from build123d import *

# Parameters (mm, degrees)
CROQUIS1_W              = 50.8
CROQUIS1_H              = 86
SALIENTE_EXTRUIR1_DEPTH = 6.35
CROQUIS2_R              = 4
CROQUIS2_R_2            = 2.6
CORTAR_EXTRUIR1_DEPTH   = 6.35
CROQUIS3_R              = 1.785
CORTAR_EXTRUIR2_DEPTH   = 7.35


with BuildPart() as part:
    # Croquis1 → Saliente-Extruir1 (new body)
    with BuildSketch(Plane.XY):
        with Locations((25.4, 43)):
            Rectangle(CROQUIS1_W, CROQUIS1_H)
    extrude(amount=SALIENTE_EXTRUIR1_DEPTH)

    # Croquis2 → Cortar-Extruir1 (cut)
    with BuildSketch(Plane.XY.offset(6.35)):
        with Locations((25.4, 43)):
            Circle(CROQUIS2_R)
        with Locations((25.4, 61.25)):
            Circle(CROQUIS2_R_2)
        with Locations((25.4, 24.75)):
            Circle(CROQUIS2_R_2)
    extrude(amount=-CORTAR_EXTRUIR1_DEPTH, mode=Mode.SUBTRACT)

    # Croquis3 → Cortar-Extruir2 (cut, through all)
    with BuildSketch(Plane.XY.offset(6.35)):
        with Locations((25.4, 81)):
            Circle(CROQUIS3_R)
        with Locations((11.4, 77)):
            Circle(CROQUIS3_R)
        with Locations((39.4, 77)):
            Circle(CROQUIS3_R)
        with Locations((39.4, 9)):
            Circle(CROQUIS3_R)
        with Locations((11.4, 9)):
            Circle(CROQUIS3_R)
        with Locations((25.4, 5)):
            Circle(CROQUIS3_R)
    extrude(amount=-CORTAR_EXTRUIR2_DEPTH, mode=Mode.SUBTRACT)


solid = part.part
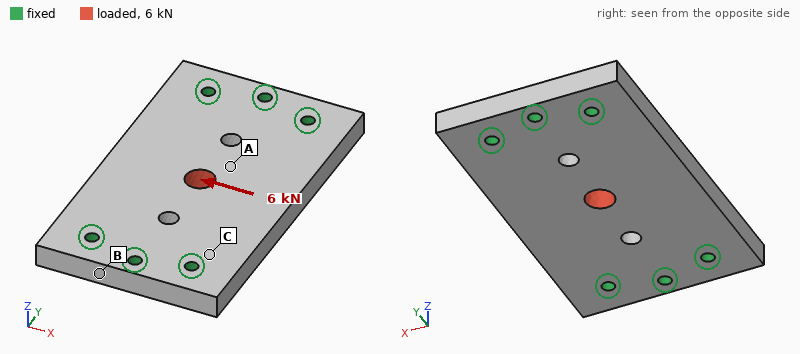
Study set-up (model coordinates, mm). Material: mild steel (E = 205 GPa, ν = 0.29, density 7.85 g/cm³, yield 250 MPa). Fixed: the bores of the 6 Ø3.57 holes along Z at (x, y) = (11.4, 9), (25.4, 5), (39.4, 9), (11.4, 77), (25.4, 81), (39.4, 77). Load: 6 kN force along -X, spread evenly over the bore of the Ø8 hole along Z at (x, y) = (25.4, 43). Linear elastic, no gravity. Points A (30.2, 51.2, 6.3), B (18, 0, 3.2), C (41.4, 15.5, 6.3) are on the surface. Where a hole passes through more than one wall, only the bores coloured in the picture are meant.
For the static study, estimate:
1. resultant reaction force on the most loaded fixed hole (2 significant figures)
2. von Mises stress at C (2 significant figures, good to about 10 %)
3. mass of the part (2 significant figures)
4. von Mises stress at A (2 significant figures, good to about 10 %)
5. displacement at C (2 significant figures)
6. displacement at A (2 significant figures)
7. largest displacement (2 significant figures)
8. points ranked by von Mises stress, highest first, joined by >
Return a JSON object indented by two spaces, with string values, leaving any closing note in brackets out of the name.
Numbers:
{
  "resultant reaction force on the most loaded fixed hole": "1.8 kN",
  "von Mises stress at C": "14 MPa",
  "mass of the part": "210 g",
  "von Mises stress at A": "24 MPa",
  "displacement at C": "1.4 µm",
  "displacement at A": "5.3 µm",
  "largest displacement": "6.9 µm",
  "points ranked by von Mises stress, highest first, joined by >": "A > C > B"
}
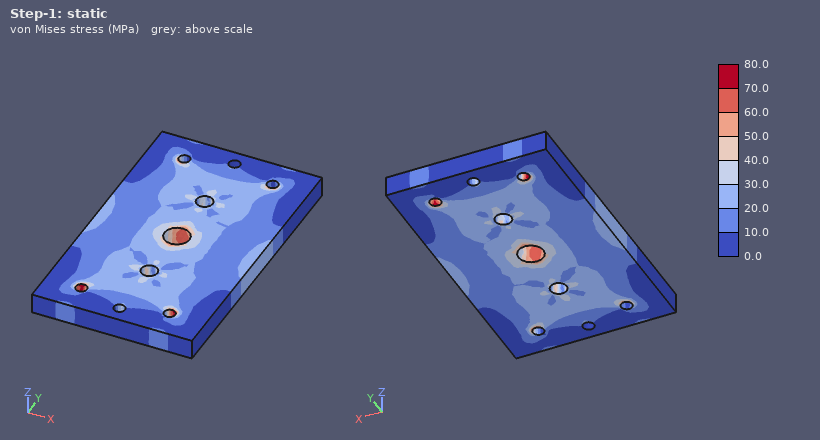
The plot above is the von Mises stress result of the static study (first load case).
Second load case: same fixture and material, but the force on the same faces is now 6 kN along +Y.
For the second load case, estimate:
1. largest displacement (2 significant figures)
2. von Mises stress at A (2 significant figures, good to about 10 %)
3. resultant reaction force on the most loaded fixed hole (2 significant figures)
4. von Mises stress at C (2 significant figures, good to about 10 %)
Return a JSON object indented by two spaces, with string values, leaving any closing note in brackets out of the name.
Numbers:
{
  "largest displacement": "3.3 µm",
  "von Mises stress at A": "26 MPa",
  "resultant reaction force on the most loaded fixed hole": "1.2 kN",
  "von Mises stress at C": "12 MPa"
}
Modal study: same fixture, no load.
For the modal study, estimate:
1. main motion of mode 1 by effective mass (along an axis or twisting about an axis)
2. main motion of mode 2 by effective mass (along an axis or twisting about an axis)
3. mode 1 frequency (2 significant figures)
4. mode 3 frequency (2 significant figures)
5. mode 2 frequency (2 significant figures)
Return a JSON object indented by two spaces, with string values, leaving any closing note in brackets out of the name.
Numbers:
{
  "main motion of mode 1 by effective mass": "along Z",
  "main motion of mode 2 by effective mass": "twisting about Y",
  "mode 1 frequency": "6400 Hz",
  "mode 3 frequency": "16 kHz",
  "mode 2 frequency": "8100 Hz"
}
